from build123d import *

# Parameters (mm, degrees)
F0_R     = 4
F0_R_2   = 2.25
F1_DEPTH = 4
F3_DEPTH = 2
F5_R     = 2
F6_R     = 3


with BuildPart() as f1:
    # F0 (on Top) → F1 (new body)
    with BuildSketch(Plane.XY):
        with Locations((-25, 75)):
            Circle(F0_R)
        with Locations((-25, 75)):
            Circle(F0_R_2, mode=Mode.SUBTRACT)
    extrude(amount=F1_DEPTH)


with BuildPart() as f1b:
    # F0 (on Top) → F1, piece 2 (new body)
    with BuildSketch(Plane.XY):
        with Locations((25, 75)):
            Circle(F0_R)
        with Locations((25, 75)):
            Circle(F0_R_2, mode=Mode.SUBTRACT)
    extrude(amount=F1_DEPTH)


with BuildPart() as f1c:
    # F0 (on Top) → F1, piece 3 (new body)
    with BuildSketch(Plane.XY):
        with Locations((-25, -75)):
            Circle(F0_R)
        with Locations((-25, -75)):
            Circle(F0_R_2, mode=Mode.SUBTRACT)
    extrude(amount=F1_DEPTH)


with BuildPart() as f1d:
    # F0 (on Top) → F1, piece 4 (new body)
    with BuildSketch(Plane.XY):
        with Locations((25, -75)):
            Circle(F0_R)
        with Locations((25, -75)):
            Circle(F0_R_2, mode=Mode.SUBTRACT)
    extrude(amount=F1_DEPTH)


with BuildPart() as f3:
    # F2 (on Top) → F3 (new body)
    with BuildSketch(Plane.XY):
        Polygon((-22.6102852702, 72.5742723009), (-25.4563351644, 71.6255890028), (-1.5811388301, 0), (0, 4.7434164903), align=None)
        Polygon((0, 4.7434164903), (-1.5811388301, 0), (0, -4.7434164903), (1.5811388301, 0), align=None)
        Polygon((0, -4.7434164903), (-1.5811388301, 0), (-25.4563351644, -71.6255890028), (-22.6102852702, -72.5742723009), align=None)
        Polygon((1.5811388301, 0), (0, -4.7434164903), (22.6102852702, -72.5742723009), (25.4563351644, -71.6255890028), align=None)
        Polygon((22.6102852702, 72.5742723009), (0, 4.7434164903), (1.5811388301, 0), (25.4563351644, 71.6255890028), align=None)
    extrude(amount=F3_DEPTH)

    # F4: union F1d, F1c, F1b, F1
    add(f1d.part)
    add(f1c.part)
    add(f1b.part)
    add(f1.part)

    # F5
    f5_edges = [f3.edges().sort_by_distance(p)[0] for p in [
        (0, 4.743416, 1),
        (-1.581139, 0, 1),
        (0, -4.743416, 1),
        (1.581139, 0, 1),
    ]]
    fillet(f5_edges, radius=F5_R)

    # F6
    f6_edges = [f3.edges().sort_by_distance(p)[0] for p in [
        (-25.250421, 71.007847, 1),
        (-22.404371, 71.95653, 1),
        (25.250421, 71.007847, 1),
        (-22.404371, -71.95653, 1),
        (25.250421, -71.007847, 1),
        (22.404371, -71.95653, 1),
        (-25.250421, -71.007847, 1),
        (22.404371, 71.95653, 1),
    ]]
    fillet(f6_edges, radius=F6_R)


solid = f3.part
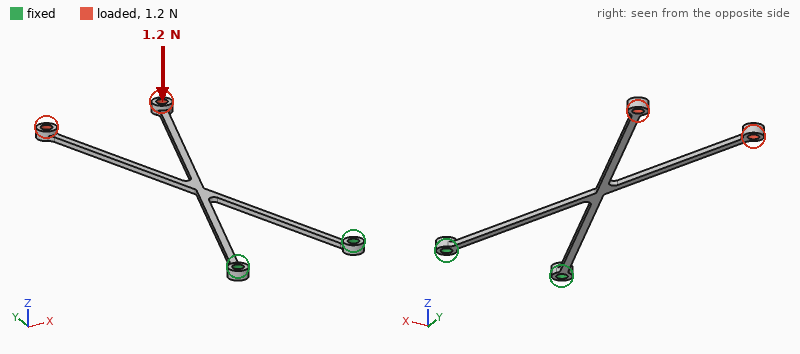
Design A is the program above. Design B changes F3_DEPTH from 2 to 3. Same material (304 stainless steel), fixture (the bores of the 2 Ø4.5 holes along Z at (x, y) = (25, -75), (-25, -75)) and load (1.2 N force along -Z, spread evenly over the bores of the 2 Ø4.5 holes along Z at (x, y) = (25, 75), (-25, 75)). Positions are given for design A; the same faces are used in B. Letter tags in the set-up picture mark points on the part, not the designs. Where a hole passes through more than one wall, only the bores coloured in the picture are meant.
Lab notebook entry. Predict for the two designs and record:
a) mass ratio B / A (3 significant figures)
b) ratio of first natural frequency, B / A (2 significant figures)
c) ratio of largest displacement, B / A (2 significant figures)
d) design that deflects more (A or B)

1.38
1.6
0.30
A
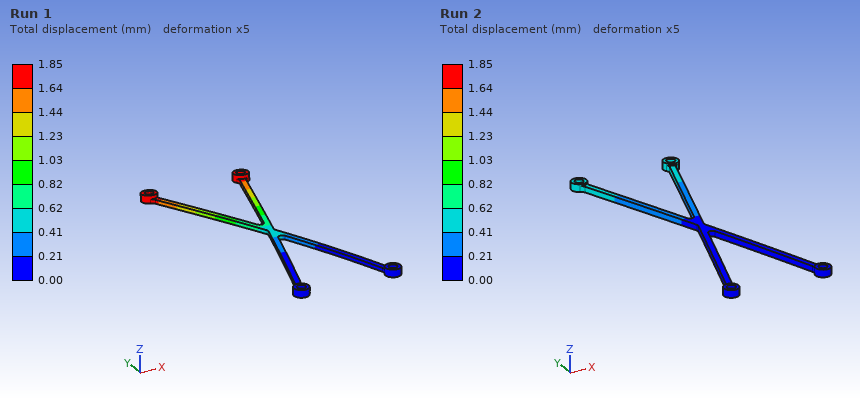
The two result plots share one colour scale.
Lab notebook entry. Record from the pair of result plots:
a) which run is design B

Run 2
